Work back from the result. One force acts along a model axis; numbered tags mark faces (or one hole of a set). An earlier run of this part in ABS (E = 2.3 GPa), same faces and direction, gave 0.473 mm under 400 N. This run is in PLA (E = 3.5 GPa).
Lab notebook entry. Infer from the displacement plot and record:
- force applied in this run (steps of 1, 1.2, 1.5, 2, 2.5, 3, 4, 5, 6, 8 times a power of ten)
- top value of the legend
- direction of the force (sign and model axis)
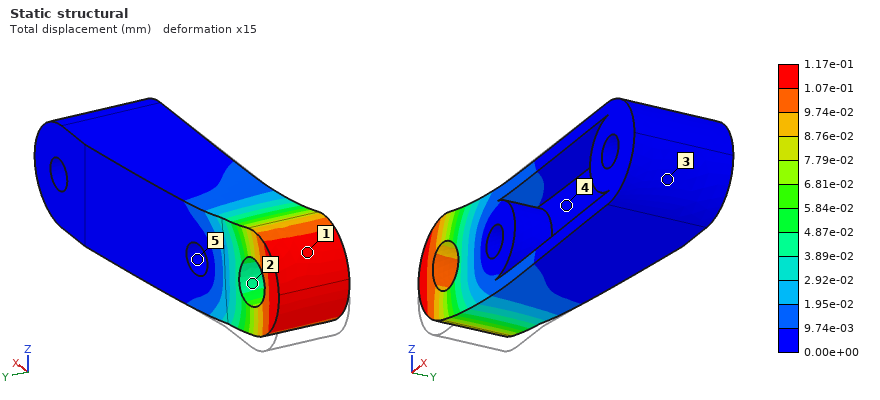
150 N
1.17e-01 mm
+Z
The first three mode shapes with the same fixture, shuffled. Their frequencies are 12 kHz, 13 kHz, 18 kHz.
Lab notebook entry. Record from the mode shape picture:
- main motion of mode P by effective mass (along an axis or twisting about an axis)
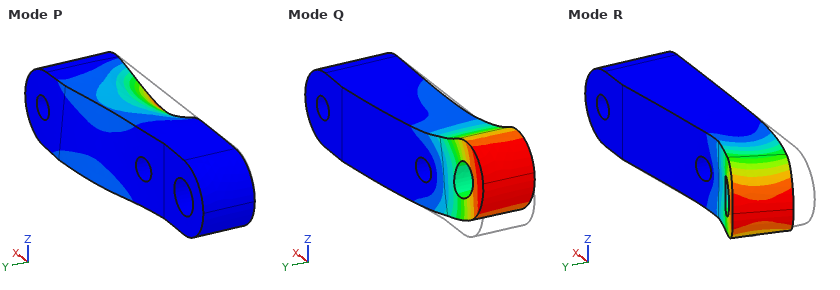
along Z
